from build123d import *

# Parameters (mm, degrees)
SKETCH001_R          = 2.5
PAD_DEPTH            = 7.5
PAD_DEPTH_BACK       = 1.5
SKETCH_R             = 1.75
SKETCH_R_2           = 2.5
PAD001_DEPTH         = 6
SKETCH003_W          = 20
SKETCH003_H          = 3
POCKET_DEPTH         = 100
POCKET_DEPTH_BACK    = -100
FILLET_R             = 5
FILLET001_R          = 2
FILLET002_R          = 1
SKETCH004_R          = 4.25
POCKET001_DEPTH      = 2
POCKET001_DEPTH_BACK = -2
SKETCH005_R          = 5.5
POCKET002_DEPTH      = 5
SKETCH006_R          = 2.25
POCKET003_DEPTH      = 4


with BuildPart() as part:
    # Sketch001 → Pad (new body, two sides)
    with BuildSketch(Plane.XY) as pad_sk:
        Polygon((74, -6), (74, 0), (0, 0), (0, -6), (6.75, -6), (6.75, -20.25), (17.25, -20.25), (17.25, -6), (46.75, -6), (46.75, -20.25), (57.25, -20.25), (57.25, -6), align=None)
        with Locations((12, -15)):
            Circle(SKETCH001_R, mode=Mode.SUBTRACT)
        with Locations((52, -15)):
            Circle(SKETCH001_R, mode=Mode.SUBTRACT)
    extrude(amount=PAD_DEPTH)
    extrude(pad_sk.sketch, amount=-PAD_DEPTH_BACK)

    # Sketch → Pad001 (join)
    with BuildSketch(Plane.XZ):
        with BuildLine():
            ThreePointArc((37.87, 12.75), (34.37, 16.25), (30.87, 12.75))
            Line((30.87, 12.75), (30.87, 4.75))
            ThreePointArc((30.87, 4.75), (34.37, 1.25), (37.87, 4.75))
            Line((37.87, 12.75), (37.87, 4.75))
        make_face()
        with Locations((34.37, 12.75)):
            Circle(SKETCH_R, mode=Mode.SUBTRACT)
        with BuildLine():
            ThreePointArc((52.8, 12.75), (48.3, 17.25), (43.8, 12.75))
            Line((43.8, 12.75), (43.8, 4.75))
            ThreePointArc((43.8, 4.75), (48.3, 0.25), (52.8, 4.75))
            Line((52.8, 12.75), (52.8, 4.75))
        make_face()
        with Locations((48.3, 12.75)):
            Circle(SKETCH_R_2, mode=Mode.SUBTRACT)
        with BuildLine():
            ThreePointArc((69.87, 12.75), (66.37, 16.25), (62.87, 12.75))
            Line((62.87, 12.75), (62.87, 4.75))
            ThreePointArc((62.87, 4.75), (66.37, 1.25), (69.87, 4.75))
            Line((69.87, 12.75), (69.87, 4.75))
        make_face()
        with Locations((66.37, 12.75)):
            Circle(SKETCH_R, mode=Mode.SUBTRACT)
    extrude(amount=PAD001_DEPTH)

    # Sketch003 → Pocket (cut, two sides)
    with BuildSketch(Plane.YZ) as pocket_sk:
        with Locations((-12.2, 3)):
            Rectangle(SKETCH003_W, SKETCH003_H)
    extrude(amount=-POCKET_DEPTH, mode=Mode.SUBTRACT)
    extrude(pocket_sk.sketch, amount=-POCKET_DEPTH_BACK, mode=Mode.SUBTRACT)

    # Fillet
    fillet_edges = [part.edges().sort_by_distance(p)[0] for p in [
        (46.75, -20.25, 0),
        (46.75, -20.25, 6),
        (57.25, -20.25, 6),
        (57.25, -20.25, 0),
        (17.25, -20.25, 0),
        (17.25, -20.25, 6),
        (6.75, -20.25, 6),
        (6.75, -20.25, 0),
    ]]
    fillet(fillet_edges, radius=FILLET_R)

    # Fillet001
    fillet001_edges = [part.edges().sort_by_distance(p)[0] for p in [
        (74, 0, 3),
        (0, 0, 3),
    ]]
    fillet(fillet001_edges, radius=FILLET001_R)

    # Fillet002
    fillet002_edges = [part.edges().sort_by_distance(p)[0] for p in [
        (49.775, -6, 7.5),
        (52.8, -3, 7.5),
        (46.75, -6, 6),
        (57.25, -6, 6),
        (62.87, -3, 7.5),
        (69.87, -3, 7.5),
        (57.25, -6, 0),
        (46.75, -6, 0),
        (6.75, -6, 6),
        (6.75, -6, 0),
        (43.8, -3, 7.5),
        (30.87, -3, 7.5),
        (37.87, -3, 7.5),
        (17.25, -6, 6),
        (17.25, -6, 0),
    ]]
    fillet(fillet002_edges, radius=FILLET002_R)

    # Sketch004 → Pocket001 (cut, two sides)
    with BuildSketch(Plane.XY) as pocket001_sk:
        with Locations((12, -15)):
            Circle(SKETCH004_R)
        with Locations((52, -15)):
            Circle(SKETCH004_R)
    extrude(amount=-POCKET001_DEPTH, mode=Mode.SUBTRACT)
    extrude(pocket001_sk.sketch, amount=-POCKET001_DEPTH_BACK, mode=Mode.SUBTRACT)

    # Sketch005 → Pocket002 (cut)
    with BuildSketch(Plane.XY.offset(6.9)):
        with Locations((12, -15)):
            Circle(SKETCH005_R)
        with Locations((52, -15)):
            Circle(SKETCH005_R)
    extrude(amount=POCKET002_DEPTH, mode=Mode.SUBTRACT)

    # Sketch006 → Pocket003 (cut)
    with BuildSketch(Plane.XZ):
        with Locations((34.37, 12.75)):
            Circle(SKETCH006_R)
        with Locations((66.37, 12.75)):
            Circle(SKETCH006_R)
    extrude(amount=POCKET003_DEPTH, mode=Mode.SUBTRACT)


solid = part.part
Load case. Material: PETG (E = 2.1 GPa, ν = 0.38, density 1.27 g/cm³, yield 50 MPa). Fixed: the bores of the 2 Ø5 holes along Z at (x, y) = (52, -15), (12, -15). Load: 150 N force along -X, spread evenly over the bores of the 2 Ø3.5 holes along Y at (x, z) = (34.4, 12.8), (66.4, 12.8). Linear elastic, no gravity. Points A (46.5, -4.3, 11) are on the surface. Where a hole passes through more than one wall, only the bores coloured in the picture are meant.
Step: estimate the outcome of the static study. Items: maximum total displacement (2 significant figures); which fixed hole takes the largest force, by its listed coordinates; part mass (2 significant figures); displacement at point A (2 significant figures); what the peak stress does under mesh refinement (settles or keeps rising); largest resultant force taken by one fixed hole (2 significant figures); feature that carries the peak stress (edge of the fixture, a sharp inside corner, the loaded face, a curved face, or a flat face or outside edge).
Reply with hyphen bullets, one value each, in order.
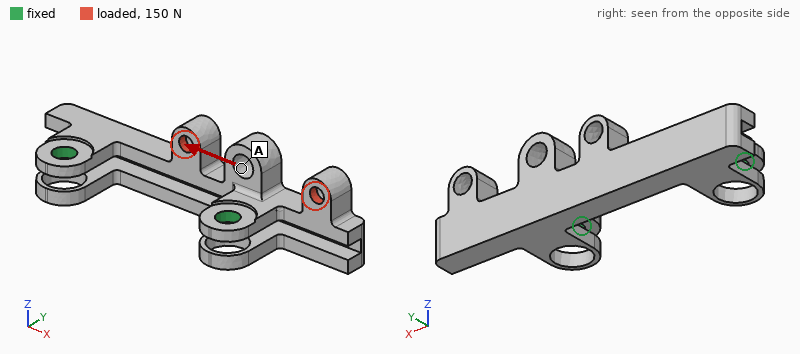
- 0.87 mm
- (52, -15)
- 6.5 g
- 0.22 mm
- keeps rising
- 100 N
- edge of the fixture
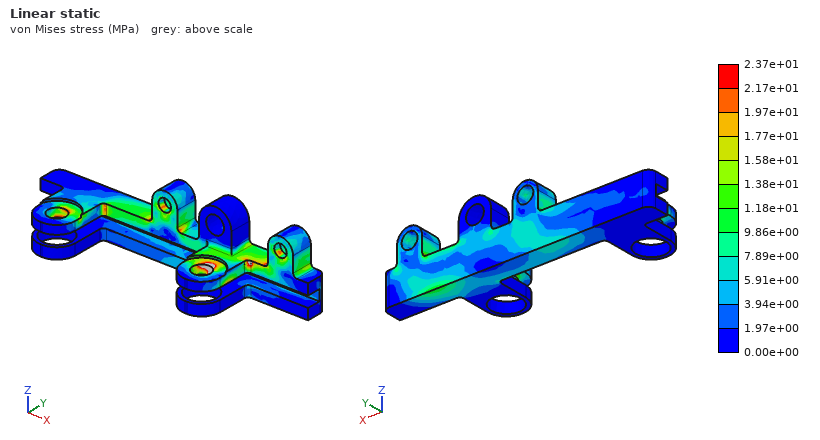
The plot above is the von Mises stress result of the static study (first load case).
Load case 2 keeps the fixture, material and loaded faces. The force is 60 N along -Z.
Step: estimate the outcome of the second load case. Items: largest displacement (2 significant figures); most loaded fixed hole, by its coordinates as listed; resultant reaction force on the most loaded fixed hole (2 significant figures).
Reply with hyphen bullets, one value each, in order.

- 0.87 mm
- (52, -15)
- 55 N
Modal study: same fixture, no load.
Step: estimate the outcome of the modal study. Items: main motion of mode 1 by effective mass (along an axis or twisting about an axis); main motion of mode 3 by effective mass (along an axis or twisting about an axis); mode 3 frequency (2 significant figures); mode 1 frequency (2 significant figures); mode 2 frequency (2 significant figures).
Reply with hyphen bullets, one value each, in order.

- along Z
- along Z
- 1600 Hz
- 690 Hz
- 1000 Hz
